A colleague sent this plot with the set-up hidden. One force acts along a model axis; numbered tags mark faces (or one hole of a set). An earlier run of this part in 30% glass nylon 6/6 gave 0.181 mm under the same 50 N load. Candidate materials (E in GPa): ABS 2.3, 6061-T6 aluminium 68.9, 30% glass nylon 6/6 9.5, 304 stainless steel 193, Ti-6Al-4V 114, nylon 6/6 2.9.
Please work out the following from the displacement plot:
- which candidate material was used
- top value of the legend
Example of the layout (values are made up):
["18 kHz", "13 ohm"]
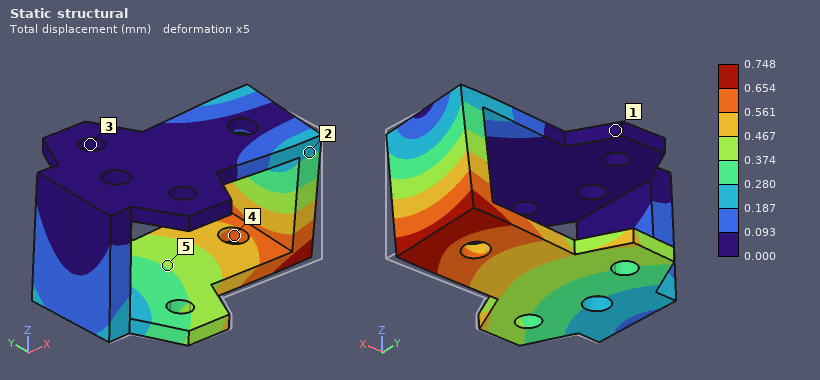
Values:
["ABS", "0.748 mm"]
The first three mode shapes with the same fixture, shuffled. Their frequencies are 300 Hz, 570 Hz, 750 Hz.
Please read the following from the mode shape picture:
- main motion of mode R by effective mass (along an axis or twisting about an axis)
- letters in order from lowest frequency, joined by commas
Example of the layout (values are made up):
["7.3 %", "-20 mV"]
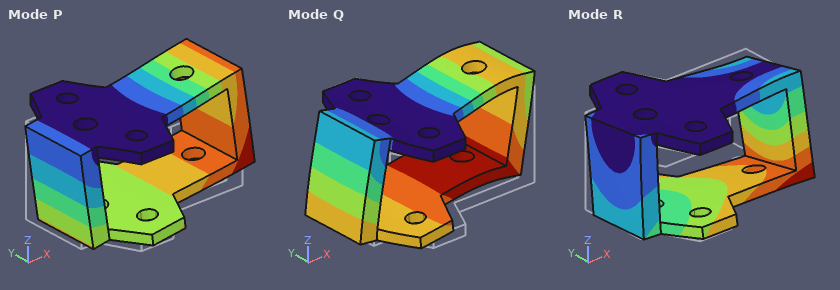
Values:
["along Y", "P, R, Q"]
